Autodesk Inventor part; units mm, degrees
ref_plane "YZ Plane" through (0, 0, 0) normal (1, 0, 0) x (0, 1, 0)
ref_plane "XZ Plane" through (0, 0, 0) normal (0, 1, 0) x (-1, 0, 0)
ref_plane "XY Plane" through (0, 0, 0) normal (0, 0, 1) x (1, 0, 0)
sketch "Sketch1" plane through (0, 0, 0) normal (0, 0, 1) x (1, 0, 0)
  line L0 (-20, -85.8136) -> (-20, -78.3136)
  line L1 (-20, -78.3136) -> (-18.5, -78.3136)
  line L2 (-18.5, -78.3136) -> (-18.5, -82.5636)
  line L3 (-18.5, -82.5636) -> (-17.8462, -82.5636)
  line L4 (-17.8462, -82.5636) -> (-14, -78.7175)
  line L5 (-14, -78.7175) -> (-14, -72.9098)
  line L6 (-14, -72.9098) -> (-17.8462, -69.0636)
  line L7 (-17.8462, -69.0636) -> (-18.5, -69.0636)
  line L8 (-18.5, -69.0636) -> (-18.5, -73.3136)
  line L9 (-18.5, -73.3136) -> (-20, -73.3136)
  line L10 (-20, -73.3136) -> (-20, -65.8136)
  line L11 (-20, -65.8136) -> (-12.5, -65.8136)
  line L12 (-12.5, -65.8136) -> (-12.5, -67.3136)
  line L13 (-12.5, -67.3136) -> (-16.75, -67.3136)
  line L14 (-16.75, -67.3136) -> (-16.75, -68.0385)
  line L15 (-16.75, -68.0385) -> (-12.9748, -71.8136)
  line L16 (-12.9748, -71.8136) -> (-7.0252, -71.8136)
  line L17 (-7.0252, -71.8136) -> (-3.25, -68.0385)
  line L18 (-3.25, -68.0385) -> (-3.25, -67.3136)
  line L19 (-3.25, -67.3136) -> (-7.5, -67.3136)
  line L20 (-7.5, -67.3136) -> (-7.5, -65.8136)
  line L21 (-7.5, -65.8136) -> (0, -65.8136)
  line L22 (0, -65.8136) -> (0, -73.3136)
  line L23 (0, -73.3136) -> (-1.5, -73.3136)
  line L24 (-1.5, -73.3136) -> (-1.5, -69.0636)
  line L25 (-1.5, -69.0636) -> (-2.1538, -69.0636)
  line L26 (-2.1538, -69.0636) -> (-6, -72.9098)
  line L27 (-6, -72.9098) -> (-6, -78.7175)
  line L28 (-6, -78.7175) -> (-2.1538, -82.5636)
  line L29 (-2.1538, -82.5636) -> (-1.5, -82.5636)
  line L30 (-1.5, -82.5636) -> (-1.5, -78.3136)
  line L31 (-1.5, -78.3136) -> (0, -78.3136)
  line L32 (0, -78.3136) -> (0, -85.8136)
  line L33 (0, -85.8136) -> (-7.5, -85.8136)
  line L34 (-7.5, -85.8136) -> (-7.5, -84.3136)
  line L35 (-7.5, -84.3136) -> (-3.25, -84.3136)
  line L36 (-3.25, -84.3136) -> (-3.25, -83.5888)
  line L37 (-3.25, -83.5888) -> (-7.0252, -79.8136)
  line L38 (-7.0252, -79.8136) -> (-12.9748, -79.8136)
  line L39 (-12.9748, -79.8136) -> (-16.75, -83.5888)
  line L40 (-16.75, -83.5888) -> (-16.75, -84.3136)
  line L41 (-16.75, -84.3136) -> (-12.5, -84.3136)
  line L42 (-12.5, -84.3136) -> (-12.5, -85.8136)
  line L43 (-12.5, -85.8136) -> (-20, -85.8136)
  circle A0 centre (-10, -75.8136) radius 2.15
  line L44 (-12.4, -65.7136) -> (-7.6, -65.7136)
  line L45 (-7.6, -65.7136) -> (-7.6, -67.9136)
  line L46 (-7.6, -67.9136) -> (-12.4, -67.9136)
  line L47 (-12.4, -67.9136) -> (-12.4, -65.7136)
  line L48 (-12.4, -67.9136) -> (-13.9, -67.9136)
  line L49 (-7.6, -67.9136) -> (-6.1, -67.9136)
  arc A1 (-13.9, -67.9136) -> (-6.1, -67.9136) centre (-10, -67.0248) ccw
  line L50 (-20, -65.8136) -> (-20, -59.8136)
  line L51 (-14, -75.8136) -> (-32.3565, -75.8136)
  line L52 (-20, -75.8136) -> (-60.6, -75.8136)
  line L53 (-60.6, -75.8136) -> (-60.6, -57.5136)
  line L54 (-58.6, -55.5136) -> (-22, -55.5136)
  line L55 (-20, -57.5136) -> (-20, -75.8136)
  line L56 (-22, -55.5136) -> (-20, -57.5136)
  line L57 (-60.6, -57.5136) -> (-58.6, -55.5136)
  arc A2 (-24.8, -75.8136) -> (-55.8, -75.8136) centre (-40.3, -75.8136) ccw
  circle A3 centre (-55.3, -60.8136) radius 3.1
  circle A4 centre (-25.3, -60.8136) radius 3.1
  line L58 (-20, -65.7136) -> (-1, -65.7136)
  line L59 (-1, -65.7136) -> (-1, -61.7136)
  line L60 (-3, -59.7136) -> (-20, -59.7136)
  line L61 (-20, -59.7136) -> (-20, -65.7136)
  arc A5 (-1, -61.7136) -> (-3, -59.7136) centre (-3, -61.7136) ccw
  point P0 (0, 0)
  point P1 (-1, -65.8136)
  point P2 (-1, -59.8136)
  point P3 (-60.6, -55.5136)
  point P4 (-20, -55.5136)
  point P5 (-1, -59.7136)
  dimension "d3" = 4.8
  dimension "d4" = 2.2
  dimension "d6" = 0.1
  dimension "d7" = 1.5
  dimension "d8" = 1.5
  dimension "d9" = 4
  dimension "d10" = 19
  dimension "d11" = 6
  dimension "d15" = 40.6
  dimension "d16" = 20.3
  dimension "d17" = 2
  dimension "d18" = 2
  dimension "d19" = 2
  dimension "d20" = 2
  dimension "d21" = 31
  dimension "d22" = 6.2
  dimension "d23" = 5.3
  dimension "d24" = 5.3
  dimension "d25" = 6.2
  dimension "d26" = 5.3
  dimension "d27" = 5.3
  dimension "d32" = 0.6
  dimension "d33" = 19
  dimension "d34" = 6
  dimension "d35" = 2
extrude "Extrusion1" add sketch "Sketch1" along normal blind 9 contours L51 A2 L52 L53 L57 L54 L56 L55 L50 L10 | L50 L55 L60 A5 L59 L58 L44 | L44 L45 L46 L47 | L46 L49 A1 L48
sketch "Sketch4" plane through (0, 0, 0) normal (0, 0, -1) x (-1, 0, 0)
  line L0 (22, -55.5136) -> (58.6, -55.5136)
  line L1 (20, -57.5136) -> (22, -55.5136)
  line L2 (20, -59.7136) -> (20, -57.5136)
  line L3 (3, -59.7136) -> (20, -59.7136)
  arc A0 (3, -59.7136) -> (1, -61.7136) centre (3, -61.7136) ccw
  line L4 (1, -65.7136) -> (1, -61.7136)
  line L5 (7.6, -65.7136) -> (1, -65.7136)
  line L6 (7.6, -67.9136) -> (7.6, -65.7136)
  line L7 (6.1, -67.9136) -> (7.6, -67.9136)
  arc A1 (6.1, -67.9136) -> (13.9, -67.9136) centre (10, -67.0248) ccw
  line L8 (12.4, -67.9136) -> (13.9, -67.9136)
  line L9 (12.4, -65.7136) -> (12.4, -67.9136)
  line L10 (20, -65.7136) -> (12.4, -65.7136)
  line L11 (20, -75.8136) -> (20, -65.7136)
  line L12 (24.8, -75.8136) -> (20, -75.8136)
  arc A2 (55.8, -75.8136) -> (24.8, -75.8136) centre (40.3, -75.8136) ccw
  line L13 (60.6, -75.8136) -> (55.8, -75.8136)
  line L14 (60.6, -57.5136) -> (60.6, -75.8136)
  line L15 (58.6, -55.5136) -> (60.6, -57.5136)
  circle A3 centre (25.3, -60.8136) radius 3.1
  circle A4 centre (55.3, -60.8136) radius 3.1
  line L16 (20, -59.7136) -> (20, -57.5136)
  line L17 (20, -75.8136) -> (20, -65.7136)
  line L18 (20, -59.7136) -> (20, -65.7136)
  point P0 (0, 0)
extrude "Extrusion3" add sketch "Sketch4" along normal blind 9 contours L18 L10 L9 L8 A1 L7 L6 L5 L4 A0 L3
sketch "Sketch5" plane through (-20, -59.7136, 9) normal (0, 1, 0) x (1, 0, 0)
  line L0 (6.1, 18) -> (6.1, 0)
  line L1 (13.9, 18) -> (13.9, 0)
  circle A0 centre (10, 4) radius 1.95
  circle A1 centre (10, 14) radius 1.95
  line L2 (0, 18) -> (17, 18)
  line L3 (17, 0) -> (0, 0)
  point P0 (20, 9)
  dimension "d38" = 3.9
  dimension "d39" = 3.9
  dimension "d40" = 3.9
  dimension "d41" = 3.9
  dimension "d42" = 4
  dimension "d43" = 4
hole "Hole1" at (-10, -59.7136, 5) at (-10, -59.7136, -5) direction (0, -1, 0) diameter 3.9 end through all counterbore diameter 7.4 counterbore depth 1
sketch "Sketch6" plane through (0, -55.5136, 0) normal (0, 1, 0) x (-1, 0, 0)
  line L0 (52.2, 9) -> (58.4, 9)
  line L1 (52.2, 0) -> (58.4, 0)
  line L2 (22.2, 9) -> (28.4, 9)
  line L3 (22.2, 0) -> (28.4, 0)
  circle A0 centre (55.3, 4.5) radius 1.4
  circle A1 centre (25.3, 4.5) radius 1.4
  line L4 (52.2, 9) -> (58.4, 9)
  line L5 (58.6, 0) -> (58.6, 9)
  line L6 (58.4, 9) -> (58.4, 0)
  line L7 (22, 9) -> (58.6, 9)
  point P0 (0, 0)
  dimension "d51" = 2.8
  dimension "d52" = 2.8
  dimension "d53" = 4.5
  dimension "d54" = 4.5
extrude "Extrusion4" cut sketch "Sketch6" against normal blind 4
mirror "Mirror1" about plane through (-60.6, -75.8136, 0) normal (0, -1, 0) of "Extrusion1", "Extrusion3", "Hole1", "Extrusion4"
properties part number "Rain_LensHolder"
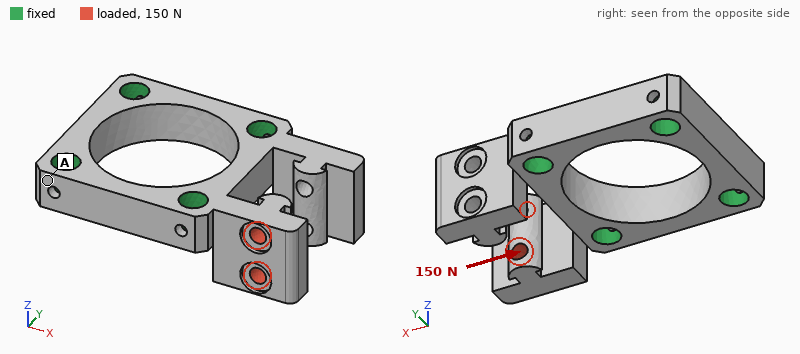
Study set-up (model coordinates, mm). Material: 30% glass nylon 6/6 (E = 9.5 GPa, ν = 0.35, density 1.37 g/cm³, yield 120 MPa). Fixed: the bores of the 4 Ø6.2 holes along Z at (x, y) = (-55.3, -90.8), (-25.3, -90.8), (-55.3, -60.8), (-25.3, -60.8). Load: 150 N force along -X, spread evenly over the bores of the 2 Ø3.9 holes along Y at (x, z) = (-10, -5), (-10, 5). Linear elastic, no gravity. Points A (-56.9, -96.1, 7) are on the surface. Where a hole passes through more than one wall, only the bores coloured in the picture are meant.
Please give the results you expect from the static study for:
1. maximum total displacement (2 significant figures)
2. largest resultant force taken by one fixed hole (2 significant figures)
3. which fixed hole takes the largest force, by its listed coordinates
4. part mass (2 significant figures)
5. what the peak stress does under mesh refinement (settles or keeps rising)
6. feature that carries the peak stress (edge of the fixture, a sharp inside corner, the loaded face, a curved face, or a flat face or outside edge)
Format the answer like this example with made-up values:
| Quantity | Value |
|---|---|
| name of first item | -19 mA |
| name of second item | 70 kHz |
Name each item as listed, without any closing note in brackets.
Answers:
| Quantity | Value |
|---|---|
| maximum total displacement | 63 µm |
| largest resultant force taken by one fixed hole | 150 N |
| which fixed hole takes the largest force, by its listed coordinates | (-25.3, -90.8) |
| part mass | 15 g |
| what the peak stress does under mesh refinement | keeps rising |
| feature that carries the peak stress | a sharp inside corner |
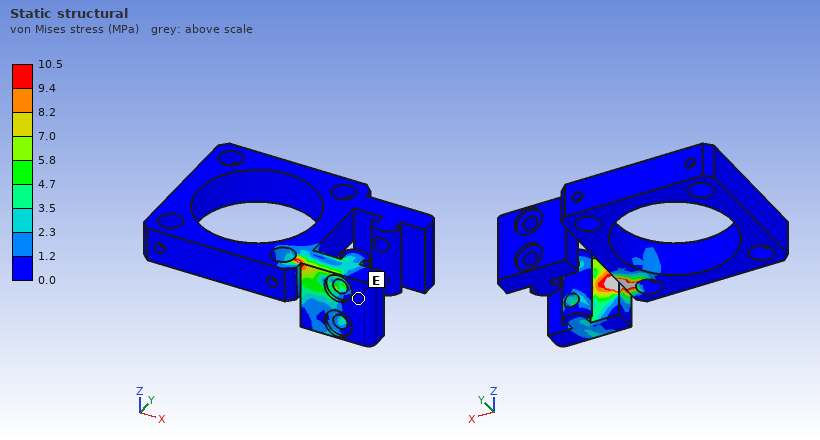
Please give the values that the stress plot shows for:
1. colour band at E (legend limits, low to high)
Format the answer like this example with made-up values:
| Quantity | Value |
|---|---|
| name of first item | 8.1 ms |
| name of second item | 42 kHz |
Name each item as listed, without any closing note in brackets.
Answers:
| Quantity | Value |
|---|---|
| colour band at E | 0.0 to 1.2 MPa |
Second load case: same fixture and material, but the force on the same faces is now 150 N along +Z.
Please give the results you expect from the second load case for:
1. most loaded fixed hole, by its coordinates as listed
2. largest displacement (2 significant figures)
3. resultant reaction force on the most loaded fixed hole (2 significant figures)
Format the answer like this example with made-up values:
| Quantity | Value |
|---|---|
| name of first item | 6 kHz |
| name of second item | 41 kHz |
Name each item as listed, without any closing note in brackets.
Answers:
| Quantity | Value |
|---|---|
| most loaded fixed hole, by its coordinates as listed | (-25.3, -90.8) |
| largest displacement | 81 µm |
| resultant reaction force on the most loaded fixed hole | 150 N |
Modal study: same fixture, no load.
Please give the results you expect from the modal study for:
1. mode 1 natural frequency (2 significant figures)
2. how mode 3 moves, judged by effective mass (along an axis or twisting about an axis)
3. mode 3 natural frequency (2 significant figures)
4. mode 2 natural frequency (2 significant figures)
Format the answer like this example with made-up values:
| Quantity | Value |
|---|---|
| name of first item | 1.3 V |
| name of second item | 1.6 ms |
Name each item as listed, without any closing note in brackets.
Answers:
| Quantity | Value |
|---|---|
| mode 1 natural frequency | 3800 Hz |
| how mode 3 moves, judged by effective mass | along Z |
| mode 3 natural frequency | 4800 Hz |
| mode 2 natural frequency | 3800 Hz |
